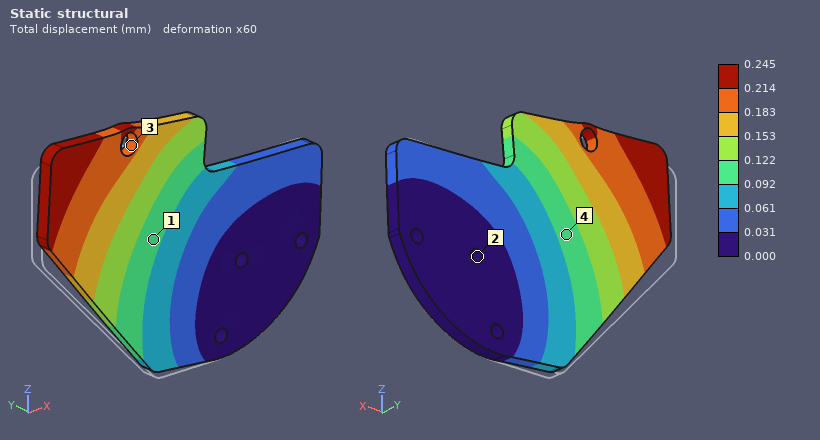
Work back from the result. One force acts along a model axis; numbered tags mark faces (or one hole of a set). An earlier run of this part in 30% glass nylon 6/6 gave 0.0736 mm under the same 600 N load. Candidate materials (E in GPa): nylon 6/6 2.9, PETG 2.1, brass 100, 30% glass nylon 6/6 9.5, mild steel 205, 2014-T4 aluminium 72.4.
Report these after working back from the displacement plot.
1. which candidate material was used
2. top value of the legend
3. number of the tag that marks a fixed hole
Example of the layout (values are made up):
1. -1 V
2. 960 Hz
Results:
1. nylon 6/6
2. 0.245 mm
3. 2
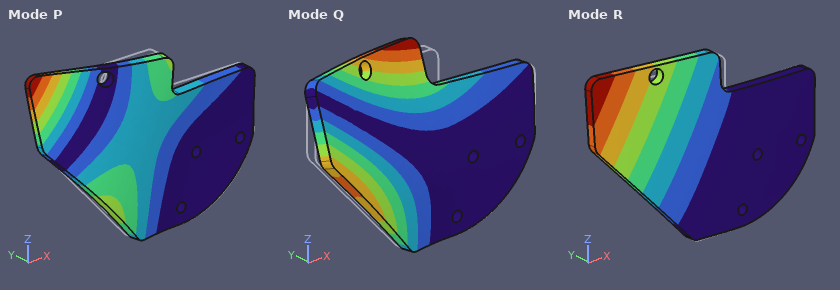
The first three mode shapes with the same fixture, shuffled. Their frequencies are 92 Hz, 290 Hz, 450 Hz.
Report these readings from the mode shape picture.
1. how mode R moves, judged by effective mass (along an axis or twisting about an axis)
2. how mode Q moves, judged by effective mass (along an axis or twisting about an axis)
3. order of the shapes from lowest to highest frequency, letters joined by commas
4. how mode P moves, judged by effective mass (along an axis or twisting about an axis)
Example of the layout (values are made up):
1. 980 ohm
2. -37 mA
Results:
1. along Y
2. twisting about X
3. R, Q, P
4. along Y
